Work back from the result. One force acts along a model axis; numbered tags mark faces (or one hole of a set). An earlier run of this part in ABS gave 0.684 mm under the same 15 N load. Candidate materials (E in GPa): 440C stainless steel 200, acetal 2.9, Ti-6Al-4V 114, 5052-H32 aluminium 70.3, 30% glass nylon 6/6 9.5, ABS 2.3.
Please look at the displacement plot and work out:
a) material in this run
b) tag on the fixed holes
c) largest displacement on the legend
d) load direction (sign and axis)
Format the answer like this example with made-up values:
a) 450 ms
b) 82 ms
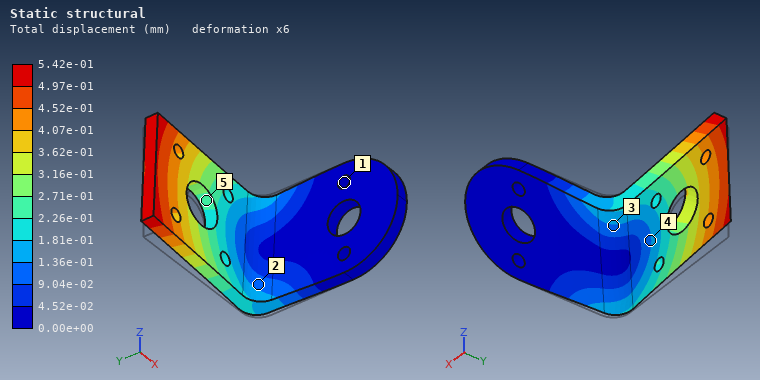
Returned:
a) acetal
b) 1
c) 5.42e-01 mm
d) +Z
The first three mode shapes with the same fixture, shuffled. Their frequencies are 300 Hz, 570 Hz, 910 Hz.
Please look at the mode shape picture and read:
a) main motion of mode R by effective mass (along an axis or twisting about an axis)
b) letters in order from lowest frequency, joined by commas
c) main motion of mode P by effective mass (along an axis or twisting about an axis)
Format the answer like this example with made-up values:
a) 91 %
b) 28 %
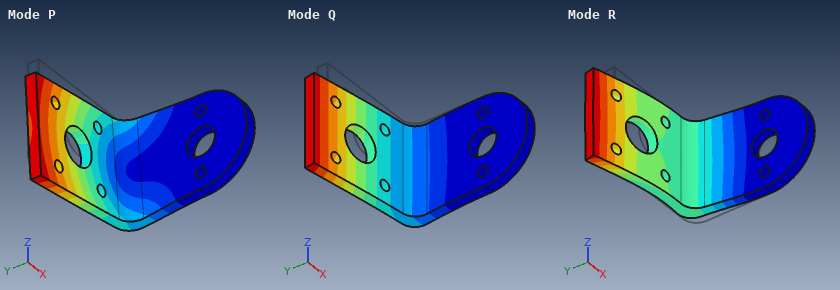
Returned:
a) along X
b) Q, P, R
c) along Z
